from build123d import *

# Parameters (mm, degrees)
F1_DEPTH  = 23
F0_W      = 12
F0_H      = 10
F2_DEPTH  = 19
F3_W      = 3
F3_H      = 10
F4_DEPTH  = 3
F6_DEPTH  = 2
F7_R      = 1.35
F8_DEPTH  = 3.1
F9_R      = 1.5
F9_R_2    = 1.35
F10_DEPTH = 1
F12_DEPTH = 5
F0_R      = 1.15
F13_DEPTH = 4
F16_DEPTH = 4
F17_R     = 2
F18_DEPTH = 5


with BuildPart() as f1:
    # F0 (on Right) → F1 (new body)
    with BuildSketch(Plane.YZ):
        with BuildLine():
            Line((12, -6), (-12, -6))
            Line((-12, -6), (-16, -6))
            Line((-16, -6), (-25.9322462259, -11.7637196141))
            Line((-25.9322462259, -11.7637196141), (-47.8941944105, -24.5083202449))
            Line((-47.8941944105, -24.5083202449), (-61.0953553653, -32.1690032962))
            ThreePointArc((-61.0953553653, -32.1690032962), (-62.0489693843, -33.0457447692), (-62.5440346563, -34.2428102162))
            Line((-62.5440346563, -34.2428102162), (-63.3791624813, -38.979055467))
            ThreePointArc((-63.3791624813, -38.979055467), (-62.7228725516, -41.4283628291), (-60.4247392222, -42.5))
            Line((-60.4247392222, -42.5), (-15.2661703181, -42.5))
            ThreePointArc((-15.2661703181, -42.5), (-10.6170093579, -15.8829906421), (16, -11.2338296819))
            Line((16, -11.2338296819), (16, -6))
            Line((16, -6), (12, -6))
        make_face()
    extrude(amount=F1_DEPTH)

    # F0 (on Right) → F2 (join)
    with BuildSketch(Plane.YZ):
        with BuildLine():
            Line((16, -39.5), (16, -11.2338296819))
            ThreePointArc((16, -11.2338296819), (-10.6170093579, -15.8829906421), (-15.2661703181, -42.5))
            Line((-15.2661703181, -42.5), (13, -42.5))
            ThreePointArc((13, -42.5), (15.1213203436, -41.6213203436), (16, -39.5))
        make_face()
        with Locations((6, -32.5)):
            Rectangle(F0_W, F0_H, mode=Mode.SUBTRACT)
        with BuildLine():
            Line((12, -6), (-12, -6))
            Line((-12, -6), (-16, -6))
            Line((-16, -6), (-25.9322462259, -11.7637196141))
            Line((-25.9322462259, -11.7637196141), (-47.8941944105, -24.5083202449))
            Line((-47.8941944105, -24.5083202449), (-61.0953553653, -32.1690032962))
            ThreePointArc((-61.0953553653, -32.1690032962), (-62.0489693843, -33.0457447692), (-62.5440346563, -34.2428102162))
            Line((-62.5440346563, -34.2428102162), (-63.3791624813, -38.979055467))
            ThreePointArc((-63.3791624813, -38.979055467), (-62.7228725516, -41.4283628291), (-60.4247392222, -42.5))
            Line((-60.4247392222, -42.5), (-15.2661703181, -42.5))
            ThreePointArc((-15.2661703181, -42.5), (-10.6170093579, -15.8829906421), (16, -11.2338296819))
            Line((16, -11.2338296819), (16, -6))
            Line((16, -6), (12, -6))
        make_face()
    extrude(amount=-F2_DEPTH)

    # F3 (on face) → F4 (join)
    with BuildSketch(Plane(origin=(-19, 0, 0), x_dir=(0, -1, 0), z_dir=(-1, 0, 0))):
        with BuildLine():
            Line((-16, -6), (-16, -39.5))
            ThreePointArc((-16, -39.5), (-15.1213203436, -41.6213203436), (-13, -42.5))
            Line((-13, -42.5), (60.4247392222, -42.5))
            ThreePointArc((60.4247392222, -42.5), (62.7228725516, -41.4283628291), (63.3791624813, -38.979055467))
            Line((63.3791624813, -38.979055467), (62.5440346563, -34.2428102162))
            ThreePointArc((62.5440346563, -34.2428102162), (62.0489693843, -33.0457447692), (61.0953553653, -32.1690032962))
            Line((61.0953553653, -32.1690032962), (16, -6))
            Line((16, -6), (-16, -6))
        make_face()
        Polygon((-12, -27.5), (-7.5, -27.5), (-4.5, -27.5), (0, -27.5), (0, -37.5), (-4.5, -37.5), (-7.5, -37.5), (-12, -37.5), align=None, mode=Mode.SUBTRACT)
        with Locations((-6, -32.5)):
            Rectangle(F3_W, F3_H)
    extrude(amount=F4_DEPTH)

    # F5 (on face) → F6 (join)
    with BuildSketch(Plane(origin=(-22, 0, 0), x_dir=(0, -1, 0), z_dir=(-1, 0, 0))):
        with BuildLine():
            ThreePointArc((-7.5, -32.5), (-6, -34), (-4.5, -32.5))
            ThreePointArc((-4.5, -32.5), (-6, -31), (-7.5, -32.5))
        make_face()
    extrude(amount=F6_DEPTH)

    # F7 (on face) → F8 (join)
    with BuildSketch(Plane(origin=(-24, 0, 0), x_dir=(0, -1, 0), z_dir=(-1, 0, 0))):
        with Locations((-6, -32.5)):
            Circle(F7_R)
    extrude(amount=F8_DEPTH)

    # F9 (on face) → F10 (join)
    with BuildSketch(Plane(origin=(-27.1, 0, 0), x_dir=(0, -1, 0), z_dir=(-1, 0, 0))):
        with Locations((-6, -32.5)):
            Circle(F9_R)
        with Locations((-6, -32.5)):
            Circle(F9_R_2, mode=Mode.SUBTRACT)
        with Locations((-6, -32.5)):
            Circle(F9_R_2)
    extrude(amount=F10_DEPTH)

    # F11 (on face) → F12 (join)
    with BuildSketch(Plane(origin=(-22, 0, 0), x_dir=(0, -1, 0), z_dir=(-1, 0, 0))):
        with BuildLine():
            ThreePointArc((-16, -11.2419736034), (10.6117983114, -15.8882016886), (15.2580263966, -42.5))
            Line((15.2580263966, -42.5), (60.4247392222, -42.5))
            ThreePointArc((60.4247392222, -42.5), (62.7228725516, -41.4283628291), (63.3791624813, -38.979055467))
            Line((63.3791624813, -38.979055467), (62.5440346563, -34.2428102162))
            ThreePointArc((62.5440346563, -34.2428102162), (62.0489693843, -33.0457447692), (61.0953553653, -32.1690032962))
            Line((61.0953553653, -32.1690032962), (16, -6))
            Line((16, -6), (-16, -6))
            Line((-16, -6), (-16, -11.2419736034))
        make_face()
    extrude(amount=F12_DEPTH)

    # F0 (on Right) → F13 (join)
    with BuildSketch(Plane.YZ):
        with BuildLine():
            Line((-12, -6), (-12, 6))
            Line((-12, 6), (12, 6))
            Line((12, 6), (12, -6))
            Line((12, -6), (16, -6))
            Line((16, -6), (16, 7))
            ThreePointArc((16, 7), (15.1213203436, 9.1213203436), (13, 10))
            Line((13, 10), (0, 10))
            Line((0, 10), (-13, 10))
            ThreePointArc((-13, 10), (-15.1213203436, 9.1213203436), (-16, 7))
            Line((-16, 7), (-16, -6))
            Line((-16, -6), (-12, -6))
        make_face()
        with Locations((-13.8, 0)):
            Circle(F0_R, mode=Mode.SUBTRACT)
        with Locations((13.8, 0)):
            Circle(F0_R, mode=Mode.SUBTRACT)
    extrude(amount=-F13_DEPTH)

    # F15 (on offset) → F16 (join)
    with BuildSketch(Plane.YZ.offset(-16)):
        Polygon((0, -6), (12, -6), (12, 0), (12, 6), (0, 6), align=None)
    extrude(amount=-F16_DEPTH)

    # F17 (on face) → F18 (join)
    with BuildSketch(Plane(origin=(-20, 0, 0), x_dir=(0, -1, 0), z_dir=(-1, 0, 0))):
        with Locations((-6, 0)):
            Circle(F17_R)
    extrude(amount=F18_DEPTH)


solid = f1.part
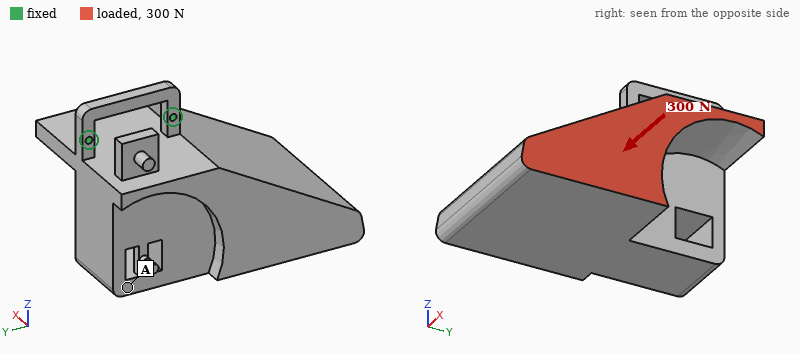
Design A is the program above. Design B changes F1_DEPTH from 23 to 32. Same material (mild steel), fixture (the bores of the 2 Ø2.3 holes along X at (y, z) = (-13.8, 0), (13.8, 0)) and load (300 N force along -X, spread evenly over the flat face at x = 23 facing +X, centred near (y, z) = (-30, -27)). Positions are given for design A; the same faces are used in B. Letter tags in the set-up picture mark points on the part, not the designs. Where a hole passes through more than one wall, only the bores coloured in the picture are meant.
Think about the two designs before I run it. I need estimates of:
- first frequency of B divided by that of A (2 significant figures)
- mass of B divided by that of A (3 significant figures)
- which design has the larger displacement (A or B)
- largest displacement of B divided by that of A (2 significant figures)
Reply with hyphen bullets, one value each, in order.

- 0.90
- 1.14
- B
- 1.1
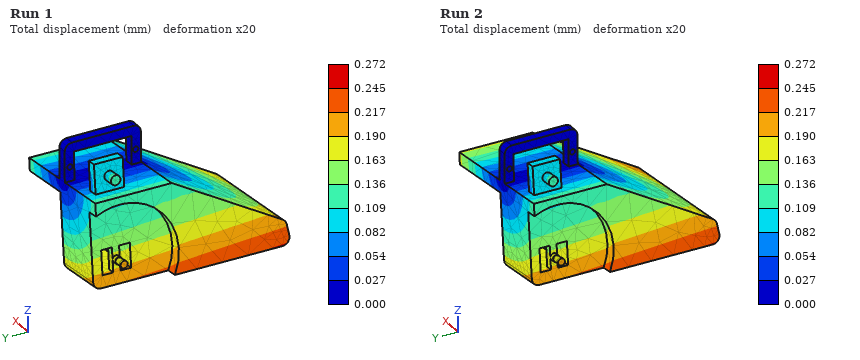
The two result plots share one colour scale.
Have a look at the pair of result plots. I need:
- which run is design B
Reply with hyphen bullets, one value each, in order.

- Run 2
